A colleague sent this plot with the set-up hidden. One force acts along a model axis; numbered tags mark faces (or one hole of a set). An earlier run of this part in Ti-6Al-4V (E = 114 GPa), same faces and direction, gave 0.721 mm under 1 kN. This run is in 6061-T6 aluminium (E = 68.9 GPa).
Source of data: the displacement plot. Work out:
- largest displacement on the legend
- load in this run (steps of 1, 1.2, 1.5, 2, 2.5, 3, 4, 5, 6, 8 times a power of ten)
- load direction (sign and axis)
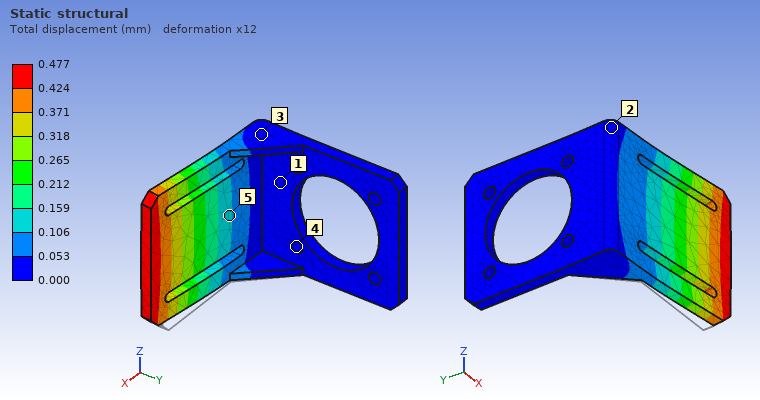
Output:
0.477 mm
400 N
-Y
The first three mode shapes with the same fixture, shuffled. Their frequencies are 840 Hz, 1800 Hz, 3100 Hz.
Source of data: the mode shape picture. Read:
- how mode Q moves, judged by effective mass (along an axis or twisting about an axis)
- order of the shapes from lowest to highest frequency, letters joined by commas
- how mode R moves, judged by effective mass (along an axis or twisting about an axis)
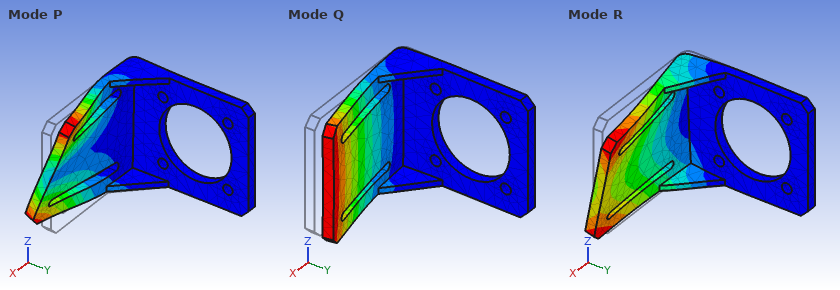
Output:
along Y
Q, R, P
along Z
